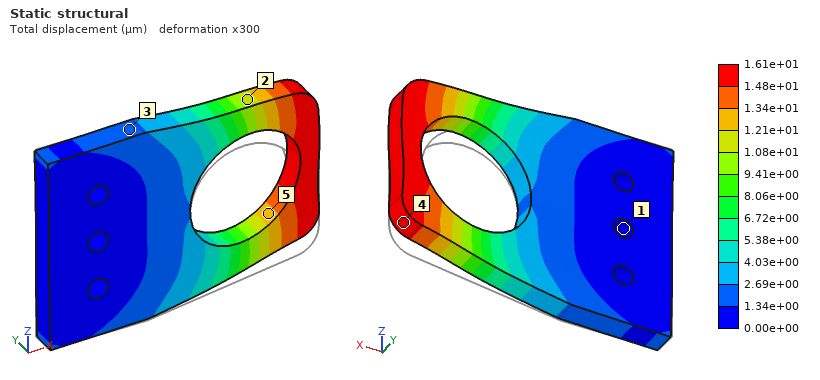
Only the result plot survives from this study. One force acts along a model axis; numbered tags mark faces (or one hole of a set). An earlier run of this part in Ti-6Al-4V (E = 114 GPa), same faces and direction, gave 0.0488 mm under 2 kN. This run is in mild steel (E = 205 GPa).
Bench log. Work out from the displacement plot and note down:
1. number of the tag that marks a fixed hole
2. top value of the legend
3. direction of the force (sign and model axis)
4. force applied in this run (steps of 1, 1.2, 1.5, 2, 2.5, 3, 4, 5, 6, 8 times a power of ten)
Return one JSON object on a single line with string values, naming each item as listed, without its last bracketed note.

{"number of the tag that marks a fixed hole": "1", "top value of the legend": "1.61e+01 µm", "direction of the force": "+Z", "force applied in this run": "1.2 kN"}
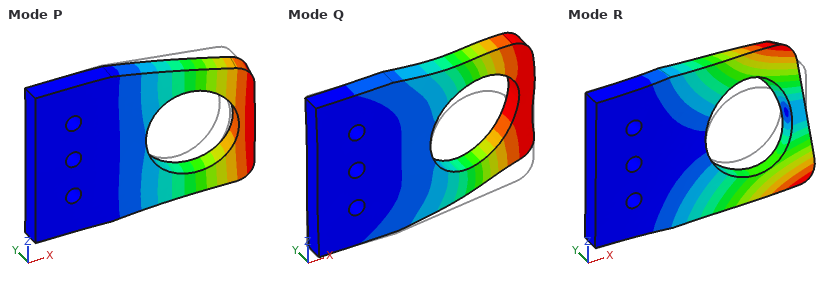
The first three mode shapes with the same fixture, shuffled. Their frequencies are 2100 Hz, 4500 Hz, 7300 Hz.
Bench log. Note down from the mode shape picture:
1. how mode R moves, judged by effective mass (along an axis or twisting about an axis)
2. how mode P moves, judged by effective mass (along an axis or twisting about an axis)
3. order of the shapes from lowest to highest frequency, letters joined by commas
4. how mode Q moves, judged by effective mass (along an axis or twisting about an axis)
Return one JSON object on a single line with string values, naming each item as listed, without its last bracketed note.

{"how mode R moves, judged by effective mass": "twisting about X", "how mode P moves, judged by effective mass": "along Y", "order of the shapes from lowest to highest frequency, letters joined by commas": "P, R, Q", "how mode Q moves, judged by effective mass": "along Z"}
